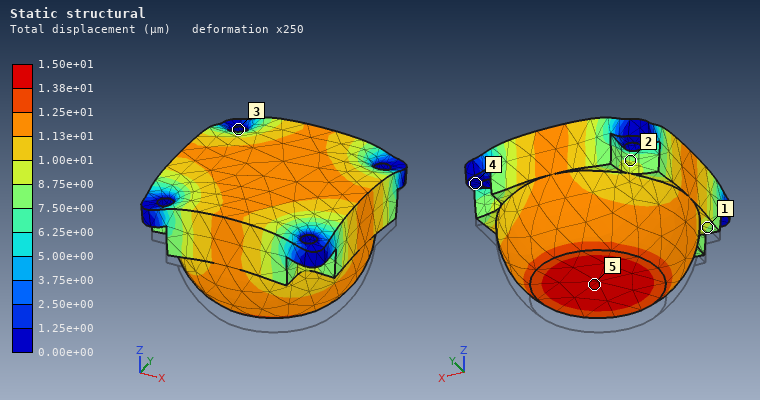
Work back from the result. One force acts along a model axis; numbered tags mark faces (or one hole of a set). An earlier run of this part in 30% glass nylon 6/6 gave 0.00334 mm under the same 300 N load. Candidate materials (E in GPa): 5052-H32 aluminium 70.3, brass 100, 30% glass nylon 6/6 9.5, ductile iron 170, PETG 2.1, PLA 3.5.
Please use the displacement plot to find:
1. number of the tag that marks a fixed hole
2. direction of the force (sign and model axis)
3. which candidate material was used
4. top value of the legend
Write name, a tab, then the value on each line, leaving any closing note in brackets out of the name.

number of the tag that marks a fixed hole	3
direction of the force	+Z
which candidate material was used	PETG
top value of the legend	1.50e+01 µm
